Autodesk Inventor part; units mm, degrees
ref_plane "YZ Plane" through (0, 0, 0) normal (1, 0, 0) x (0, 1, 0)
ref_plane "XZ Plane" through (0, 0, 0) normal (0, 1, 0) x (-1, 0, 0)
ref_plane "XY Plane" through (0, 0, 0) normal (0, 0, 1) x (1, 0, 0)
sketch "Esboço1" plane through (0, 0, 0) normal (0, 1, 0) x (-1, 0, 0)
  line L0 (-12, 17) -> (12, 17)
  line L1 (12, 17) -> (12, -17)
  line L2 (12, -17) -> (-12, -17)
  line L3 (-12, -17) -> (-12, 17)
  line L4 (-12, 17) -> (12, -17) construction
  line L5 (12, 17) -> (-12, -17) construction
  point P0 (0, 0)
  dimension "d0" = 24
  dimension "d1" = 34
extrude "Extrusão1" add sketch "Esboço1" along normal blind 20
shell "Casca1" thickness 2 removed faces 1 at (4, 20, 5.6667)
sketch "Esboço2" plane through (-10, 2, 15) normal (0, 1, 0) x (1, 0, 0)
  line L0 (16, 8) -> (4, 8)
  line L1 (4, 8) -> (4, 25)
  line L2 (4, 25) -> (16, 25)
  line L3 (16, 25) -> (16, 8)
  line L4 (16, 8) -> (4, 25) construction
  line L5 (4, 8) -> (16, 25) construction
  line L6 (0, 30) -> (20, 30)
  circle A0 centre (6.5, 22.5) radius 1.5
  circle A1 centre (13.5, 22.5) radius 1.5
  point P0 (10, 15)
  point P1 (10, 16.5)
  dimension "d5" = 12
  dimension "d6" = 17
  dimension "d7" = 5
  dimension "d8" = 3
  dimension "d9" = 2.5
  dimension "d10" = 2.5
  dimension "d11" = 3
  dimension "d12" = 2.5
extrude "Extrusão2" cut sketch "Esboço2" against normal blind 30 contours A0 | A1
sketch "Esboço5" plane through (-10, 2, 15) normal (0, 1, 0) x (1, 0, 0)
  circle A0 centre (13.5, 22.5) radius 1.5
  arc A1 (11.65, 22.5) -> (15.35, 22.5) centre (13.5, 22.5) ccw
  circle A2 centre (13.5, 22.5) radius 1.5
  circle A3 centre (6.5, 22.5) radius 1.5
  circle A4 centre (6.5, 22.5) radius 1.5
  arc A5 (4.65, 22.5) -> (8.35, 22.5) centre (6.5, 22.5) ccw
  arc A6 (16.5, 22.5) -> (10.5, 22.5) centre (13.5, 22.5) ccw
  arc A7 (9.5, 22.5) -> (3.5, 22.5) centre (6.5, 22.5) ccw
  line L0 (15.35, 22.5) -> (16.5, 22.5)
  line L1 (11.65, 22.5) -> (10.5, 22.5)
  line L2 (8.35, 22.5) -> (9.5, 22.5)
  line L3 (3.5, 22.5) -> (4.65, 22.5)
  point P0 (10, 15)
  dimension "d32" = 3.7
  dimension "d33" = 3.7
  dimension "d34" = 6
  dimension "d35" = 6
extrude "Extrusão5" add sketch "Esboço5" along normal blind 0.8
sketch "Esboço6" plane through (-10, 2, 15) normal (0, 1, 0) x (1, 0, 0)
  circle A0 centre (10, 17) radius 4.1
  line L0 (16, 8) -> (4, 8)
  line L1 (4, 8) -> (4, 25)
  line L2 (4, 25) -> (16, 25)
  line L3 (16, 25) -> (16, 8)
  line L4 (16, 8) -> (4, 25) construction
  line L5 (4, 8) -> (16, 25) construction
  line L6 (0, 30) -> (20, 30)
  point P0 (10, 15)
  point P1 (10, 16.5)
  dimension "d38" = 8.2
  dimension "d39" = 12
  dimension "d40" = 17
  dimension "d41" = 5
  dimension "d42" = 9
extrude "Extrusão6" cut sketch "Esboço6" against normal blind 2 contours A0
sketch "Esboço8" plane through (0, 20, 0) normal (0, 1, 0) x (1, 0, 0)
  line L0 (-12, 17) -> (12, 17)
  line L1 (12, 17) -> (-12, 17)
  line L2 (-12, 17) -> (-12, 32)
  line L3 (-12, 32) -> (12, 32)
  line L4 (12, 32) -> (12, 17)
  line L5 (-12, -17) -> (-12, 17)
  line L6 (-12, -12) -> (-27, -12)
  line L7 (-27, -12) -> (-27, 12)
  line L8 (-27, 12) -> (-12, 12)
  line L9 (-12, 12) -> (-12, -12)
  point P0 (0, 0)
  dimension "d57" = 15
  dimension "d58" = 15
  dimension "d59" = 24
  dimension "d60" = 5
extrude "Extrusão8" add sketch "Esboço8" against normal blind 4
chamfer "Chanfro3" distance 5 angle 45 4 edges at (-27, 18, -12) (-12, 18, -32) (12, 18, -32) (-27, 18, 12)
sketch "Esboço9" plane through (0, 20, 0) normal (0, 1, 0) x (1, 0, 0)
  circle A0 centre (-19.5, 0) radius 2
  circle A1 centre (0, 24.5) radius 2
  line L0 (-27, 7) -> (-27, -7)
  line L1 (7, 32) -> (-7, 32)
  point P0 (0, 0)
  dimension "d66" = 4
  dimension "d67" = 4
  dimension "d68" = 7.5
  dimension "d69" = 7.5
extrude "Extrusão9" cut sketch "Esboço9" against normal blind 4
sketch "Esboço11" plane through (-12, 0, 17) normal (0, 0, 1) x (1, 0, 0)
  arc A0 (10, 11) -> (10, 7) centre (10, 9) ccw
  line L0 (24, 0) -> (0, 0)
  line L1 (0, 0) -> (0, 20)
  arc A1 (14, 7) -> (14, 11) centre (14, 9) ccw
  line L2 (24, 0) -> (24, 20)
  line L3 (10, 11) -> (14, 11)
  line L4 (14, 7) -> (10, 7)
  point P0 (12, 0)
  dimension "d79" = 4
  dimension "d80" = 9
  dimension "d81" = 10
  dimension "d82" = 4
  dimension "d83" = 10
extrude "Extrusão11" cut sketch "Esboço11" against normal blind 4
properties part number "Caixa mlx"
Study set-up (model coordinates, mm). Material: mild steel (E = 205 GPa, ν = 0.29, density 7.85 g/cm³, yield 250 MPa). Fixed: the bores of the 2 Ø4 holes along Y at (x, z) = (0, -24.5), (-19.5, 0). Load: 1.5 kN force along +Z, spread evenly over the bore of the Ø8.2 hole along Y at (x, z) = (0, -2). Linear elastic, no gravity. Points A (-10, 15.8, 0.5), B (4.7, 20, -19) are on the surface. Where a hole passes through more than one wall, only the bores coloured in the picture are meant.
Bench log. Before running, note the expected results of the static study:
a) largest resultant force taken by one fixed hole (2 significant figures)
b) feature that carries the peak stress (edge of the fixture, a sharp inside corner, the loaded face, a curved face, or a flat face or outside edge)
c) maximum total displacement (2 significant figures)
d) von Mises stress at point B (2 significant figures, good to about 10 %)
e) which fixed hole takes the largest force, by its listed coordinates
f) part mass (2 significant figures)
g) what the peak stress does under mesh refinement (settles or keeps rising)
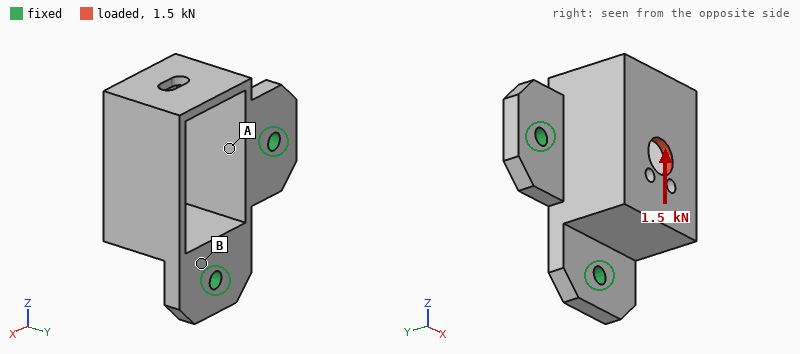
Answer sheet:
1.3 kN
edge of the fixture
0.11 mm
66 MPa
(0, -24.5)
62 g
keeps rising
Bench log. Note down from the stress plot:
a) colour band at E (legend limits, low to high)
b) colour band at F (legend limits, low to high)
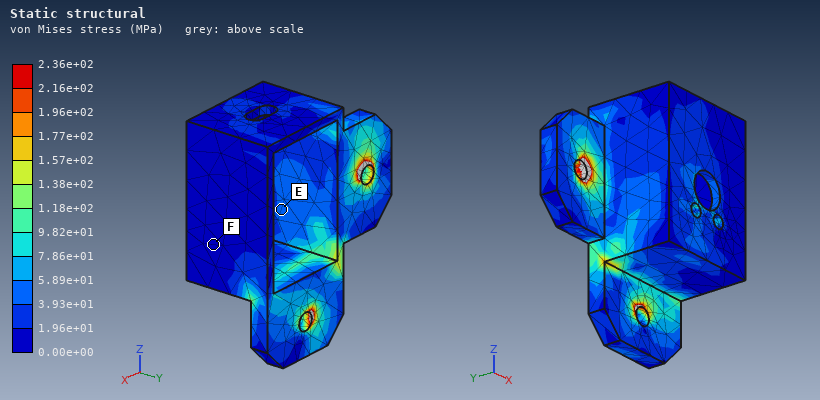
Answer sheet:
3.93e+01 to 5.89e+01 MPa
0.00e+00 to 1.96e+01 MPa
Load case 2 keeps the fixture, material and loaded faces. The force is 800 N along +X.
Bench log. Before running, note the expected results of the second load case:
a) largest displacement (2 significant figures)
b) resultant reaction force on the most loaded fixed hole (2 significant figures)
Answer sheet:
74 µm
570 N
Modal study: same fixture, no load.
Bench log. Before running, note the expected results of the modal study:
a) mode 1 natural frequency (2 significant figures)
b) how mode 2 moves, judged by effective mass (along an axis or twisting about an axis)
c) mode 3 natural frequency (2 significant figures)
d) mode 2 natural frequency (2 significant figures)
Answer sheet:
2900 Hz
along X
9200 Hz
6500 Hz
